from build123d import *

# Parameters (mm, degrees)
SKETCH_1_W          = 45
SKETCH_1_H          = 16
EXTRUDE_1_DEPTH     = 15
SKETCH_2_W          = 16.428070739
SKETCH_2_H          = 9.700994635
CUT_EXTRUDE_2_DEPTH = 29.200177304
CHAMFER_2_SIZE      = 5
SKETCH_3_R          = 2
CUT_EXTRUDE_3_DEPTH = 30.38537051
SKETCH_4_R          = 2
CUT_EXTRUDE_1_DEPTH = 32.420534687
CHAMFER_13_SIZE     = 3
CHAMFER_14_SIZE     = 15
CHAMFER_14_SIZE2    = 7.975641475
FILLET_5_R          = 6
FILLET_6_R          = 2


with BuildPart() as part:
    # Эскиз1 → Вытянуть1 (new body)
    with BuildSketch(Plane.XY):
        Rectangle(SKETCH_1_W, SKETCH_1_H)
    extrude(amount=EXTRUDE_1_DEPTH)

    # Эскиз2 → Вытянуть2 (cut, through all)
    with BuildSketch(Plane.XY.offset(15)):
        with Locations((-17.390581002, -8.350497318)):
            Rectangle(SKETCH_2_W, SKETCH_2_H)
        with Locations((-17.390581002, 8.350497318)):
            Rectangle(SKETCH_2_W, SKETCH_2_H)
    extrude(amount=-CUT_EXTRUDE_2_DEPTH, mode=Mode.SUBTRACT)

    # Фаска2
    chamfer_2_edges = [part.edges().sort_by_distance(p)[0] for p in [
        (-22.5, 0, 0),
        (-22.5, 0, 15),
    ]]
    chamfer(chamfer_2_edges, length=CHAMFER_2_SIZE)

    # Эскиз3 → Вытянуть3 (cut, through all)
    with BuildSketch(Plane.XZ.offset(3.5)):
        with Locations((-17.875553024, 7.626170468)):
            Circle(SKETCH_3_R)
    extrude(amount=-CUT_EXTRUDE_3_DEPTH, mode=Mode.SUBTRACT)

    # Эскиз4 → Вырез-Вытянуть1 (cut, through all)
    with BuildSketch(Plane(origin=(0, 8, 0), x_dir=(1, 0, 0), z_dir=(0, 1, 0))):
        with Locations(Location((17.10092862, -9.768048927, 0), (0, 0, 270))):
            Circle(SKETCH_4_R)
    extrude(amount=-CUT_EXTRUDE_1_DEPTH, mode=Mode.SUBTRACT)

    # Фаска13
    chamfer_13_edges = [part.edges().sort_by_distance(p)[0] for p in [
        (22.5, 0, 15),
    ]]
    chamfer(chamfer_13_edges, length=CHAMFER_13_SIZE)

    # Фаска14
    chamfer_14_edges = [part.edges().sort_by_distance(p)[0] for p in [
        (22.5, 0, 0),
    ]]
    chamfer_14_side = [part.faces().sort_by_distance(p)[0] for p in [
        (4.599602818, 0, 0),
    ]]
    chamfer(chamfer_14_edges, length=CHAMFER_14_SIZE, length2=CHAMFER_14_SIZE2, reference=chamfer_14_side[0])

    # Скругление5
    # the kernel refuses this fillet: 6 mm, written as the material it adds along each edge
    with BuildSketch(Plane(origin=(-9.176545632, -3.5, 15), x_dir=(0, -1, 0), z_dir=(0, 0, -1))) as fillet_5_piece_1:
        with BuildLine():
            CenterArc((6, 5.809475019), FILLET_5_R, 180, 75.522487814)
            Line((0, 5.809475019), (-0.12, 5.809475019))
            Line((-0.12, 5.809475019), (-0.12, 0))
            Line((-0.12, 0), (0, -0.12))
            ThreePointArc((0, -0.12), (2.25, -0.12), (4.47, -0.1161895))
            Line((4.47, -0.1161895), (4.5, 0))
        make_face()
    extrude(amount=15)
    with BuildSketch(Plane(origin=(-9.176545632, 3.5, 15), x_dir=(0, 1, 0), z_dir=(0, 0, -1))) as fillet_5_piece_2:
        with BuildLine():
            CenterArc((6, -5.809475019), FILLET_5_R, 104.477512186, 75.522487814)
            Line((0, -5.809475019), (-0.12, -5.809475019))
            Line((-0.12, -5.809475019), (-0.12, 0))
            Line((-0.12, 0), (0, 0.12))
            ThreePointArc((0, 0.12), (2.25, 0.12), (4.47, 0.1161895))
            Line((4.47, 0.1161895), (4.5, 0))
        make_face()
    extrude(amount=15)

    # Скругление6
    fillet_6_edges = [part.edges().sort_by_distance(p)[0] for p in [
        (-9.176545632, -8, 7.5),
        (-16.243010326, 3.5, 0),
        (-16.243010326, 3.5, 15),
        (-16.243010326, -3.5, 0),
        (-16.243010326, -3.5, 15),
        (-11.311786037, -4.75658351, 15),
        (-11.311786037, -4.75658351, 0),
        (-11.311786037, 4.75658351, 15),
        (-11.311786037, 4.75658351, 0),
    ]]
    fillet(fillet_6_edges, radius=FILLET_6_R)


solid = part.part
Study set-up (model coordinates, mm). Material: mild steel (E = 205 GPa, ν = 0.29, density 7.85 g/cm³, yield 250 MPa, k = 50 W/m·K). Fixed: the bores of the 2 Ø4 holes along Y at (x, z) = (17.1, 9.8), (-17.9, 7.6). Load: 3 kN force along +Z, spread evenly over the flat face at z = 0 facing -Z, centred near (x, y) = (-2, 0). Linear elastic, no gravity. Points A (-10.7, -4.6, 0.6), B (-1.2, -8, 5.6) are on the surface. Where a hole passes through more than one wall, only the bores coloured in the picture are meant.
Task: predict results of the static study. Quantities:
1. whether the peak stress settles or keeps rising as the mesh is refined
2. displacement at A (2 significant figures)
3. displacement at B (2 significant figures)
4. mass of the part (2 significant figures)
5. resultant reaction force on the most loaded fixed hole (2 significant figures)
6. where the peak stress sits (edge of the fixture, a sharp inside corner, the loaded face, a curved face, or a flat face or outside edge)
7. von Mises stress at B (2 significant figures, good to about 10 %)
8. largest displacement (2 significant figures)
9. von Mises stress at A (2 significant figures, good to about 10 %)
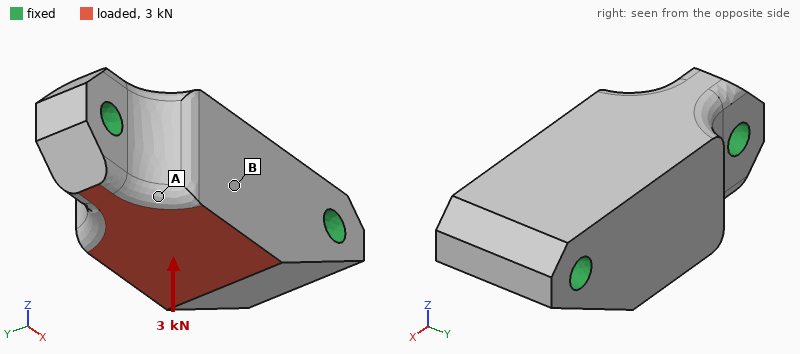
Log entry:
keeps rising
2.1 µm
3.0 µm
60 g
1.6 kN
edge of the fixture
6.4 MPa
3.2 µm
22 MPa
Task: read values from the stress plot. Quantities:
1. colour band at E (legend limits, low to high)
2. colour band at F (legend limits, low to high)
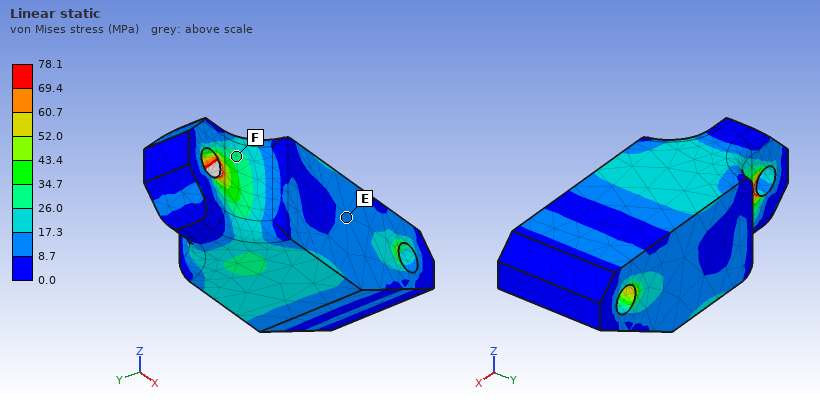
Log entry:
8.7 to 17.3 MPa
26.0 to 34.7 MPa
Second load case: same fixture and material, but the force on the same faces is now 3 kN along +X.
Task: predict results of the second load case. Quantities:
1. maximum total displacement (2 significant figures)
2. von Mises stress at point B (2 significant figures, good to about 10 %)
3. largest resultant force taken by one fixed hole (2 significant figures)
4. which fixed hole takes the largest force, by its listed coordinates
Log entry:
1.5 µm
5.2 MPa
1.8 kN
(17.1, 9.8)
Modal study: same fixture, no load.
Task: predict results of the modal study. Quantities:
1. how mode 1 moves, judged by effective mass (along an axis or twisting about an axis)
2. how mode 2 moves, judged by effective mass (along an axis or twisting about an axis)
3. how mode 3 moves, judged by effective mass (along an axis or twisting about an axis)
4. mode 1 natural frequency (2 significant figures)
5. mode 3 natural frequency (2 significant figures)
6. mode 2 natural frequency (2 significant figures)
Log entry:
along Z
along Y
along Y
26 kHz
31 kHz
28 kHz
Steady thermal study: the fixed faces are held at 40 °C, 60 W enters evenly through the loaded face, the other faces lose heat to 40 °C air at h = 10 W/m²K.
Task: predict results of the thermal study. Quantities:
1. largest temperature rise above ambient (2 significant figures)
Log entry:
65 K
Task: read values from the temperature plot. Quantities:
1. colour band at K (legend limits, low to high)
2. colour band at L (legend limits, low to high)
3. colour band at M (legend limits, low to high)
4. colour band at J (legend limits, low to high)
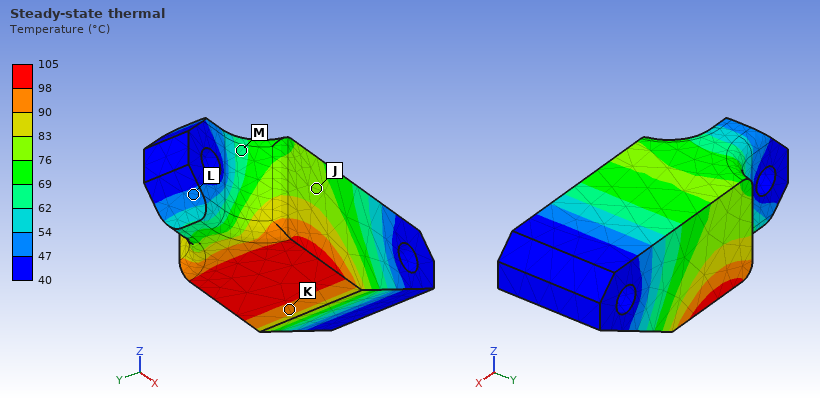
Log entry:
90 to 98 °C
47 to 54 °C
62 to 69 °C
76 to 83 °C
